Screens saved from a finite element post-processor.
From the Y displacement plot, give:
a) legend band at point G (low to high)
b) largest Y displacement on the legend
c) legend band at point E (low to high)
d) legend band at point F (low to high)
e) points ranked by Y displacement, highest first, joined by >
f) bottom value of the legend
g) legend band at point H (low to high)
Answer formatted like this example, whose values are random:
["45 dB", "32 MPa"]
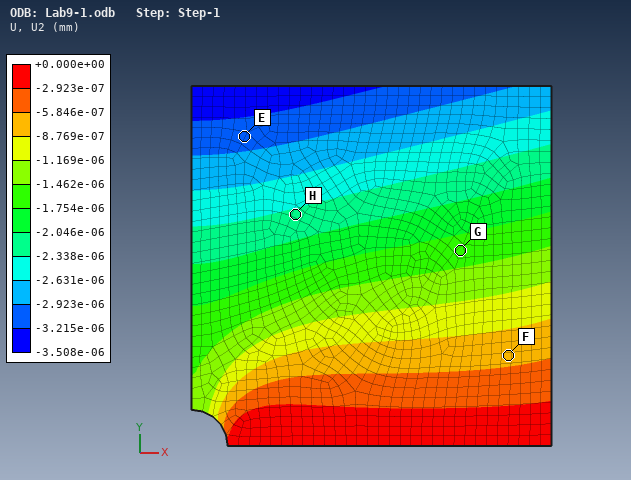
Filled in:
["-1.754e-06 to -1.462e-06 mm", "+0.000e+00 mm", "-3.215e-06 to -2.923e-06 mm", "-8.769e-07 to -5.846e-07 mm", "F > G > H > E", "-3.508e-06 mm", "-2.338e-06 to -2.046e-06 mm"]
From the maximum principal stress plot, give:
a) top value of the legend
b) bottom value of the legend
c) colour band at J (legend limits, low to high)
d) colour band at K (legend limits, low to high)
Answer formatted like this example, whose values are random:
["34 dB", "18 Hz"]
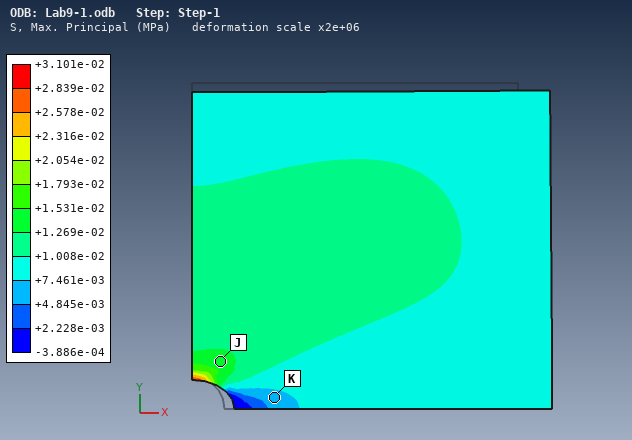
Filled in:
["+3.101e-02 MPa", "-3.886e-04 MPa", "+1.269e-02 to +1.531e-02 MPa", "+4.845e-03 to +7.461e-03 MPa"]
